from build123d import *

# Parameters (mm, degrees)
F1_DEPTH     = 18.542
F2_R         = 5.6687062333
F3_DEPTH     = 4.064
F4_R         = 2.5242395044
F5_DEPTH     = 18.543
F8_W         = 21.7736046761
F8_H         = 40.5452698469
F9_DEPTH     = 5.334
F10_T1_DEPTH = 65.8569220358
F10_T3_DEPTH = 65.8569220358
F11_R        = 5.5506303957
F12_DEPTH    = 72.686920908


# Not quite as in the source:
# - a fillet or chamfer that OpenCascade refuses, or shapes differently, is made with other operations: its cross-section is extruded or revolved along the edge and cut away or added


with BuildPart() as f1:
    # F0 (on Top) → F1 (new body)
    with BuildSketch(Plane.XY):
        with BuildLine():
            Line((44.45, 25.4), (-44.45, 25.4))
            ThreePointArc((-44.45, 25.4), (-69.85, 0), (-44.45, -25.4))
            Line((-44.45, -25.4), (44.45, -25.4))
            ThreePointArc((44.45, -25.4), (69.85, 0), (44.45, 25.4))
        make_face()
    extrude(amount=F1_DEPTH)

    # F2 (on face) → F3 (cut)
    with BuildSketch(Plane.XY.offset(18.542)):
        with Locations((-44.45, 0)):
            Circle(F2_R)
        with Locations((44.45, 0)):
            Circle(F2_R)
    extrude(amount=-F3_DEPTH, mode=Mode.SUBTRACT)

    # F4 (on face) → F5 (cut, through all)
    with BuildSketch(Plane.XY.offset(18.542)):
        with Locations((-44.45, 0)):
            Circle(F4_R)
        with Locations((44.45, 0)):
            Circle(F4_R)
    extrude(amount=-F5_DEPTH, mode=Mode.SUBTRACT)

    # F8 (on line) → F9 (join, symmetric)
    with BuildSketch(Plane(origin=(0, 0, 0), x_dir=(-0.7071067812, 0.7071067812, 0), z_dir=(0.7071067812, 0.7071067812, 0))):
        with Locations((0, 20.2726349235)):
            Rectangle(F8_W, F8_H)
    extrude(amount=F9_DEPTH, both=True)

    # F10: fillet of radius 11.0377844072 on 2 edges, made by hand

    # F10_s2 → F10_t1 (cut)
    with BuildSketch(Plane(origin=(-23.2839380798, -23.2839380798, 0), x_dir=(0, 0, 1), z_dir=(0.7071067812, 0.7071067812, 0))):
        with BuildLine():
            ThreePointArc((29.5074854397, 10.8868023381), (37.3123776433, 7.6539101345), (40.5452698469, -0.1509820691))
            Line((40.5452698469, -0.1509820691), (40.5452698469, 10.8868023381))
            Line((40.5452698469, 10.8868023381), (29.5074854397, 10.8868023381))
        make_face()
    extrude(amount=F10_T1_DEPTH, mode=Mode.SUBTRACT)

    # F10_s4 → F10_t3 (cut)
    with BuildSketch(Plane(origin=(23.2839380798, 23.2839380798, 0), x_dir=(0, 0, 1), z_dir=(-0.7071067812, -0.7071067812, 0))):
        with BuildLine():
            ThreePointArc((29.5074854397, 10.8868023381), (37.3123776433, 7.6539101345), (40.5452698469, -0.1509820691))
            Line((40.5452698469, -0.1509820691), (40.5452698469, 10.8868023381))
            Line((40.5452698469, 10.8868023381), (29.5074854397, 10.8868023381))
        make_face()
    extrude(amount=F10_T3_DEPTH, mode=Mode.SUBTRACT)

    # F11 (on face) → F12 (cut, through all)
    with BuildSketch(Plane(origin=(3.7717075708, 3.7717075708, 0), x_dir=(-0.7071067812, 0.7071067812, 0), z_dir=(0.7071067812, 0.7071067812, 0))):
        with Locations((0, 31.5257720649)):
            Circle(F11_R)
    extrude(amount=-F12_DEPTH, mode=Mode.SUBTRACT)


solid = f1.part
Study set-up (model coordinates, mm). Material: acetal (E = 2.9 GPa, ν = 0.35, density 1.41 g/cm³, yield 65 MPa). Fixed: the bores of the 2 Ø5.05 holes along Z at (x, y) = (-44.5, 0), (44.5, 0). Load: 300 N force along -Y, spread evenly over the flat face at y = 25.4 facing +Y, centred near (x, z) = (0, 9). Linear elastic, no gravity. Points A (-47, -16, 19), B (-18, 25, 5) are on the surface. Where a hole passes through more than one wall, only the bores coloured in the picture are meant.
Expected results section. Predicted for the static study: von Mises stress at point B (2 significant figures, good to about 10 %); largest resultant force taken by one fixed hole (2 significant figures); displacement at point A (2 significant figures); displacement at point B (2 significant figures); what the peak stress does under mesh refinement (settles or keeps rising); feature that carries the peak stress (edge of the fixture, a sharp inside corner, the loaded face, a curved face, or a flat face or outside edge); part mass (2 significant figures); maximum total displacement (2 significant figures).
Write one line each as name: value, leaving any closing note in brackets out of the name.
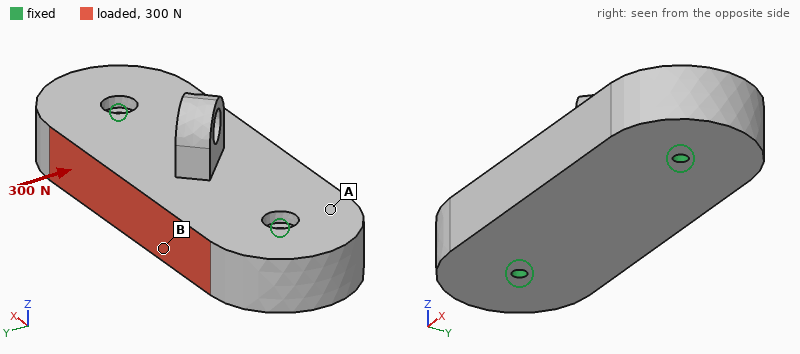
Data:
von Mises stress at point B: 0.33 MPa
largest resultant force taken by one fixed hole: 150 N
displacement at point A: 3.1 µm
displacement at point B: 8.2 µm
what the peak stress does under mesh refinement: keeps rising
feature that carries the peak stress: edge of the fixture
part mass: 170 g
maximum total displacement: 12 µm
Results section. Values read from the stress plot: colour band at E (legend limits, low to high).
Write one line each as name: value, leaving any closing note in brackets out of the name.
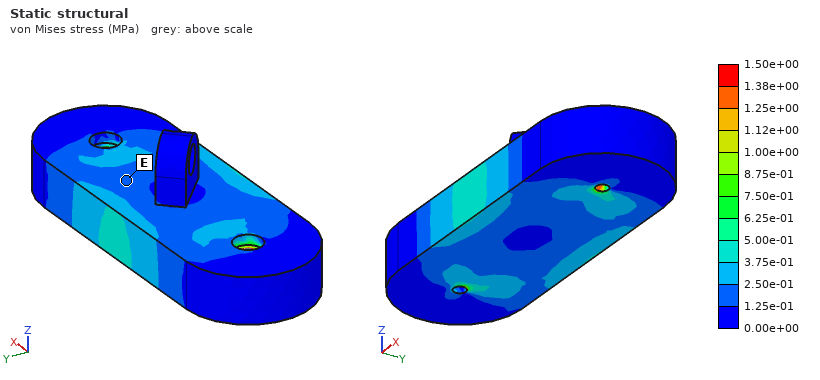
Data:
colour band at E: 1.25e-01 to 2.50e-01 MPa
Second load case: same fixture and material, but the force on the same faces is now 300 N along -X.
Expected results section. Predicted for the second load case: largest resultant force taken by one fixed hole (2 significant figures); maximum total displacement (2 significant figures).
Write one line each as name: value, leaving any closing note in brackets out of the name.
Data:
largest resultant force taken by one fixed hole: 170 N
maximum total displacement: 6.2 µm
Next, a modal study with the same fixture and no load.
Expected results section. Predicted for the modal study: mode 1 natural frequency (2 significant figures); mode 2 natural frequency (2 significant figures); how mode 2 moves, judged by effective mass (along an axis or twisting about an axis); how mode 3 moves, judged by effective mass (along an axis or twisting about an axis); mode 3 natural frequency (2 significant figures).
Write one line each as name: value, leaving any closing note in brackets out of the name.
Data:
mode 1 natural frequency: 1700 Hz
mode 2 natural frequency: 1800 Hz
how mode 2 moves, judged by effective mass: along Z
how mode 3 moves, judged by effective mass: along Y
mode 3 natural frequency: 2800 Hz
